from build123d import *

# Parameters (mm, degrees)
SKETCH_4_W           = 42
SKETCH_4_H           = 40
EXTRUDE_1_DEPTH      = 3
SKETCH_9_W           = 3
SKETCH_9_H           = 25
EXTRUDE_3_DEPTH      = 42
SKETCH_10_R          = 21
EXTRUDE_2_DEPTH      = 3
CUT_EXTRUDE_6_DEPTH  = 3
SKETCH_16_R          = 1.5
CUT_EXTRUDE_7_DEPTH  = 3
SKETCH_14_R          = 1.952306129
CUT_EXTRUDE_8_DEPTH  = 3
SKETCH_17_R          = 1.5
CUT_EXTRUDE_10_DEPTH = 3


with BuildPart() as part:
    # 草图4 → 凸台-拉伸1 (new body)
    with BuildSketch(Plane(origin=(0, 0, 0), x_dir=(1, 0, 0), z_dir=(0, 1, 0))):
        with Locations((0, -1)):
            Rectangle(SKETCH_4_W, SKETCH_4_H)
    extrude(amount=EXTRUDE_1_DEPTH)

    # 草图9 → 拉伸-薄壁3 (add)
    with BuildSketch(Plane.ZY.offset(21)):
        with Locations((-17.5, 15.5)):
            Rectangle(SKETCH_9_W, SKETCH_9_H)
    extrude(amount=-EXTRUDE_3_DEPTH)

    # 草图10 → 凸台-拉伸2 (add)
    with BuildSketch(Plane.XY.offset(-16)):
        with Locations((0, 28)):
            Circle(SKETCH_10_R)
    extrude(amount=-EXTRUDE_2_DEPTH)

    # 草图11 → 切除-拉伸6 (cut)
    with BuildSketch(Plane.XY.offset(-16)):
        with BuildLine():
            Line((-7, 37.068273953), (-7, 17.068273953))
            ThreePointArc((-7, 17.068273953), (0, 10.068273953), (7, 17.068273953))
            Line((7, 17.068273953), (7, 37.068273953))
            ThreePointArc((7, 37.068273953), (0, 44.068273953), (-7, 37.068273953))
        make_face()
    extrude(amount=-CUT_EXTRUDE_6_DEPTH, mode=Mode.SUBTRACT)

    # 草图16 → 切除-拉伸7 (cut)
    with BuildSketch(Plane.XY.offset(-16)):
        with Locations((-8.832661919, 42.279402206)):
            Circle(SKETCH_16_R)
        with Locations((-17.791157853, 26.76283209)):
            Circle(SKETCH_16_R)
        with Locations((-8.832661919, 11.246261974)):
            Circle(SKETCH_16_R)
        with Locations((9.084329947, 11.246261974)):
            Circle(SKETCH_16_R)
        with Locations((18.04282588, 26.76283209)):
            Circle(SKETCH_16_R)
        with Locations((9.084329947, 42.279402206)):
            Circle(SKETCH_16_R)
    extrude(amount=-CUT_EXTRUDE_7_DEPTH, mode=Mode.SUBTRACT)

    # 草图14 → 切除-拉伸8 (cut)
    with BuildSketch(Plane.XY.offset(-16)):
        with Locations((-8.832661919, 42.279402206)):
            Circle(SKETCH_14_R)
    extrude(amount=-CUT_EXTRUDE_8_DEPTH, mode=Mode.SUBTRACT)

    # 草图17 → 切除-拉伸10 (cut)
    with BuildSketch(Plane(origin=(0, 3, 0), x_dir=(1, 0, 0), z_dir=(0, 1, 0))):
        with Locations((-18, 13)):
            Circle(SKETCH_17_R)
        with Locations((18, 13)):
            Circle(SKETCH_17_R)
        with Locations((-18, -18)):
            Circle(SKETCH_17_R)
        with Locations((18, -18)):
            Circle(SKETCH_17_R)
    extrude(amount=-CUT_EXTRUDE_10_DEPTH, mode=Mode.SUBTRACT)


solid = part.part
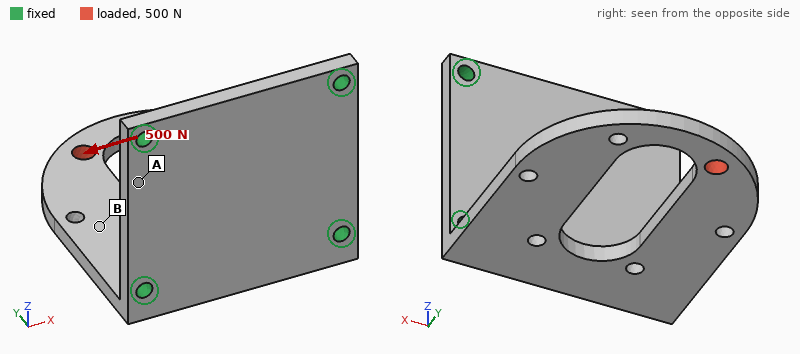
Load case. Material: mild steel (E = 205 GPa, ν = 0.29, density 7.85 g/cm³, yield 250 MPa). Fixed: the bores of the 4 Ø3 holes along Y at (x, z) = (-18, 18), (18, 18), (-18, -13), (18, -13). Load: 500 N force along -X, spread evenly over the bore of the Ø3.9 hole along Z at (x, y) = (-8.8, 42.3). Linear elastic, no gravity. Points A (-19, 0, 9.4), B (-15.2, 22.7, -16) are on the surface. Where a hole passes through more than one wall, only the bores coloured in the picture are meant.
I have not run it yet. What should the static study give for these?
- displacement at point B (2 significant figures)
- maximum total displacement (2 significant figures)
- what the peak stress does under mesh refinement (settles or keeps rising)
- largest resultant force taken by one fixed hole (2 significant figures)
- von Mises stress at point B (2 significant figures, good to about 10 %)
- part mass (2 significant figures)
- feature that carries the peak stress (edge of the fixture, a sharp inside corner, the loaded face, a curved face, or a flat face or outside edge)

14 µm
31 µm
keeps rising
620 N
26 MPa
69 g
edge of the fixture
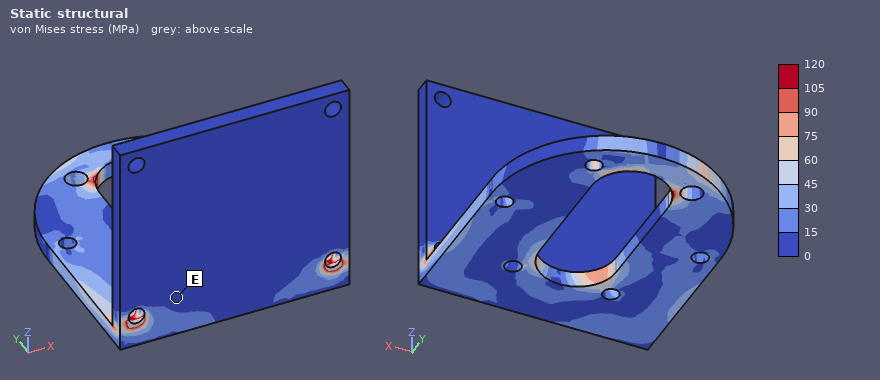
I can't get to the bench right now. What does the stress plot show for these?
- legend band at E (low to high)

0 to 15 MPa
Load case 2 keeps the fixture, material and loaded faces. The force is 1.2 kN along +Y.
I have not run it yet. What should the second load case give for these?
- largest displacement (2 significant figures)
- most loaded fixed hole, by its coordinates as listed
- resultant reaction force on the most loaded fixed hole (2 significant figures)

43 µm
(-18, -13)
930 N
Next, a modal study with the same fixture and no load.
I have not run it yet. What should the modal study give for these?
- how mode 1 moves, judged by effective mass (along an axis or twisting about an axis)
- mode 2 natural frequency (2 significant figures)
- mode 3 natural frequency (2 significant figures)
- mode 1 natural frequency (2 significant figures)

along Z
3000 Hz
6100 Hz
1200 Hz
